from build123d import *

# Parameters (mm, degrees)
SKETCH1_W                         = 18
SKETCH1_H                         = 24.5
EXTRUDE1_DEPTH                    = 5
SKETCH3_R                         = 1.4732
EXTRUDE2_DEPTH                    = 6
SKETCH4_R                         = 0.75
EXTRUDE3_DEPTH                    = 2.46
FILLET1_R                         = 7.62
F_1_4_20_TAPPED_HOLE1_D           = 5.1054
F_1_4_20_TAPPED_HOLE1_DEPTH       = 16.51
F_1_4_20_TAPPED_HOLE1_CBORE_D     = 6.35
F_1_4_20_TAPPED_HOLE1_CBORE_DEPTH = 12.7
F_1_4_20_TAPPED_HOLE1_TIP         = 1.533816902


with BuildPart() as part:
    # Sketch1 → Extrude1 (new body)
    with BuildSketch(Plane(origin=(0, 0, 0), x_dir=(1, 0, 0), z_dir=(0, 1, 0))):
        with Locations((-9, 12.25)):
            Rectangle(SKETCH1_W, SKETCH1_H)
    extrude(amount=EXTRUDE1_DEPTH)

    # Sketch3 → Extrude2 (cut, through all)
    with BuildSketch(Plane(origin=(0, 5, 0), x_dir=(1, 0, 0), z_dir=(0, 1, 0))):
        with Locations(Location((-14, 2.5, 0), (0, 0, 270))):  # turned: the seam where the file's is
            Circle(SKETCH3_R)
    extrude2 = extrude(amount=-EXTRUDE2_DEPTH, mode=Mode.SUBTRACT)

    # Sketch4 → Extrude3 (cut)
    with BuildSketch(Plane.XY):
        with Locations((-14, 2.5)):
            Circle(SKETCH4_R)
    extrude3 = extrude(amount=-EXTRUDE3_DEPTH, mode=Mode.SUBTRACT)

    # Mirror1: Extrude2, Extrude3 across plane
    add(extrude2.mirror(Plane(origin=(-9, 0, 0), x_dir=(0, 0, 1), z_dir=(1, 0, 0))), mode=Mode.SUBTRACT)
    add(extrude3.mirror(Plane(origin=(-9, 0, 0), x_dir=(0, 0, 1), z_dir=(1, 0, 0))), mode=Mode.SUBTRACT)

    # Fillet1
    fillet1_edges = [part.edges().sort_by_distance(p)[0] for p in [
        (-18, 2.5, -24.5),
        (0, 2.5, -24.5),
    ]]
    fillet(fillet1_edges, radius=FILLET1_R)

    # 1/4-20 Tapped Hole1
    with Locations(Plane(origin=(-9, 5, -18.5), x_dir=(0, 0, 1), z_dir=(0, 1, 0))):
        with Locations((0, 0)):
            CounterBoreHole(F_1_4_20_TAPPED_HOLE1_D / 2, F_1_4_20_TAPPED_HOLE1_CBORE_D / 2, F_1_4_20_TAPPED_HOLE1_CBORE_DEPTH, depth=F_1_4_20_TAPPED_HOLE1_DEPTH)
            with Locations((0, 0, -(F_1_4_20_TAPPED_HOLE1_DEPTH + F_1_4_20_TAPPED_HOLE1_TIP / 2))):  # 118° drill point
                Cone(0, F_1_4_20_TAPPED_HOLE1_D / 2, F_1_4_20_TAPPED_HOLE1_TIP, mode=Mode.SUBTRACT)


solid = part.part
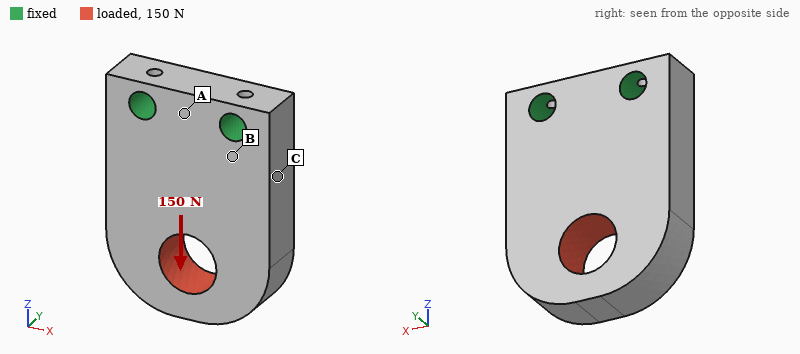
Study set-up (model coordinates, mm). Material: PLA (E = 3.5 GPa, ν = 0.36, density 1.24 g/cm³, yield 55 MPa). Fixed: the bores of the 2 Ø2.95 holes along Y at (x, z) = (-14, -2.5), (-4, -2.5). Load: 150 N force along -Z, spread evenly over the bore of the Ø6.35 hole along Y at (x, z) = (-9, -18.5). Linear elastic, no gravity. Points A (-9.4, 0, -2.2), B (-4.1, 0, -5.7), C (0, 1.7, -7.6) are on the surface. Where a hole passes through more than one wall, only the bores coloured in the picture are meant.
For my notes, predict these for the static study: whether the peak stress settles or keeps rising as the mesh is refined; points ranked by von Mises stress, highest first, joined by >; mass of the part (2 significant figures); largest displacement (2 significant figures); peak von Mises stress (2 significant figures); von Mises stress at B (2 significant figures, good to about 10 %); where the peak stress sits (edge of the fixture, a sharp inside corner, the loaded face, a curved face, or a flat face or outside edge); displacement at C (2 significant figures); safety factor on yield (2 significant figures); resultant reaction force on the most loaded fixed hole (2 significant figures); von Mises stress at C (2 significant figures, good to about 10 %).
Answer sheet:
settles
B > C > A
2.3 g
17 µm
5.5 MPa
2.4 MPa
the loaded face
3.5 µm
9.9
76 N
1.4 MPa
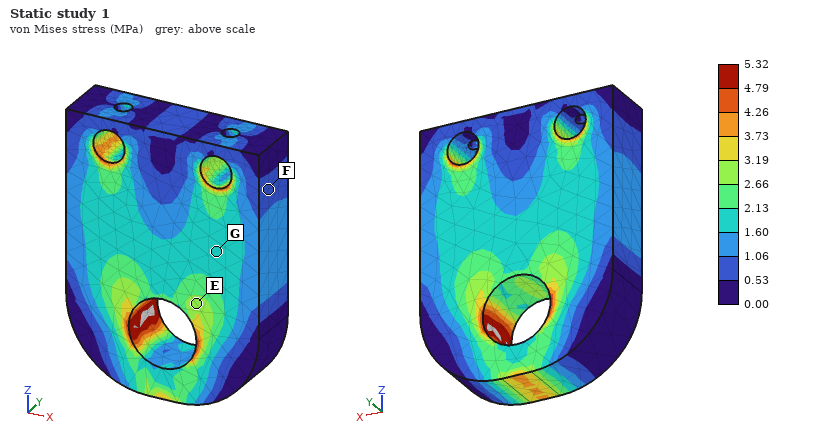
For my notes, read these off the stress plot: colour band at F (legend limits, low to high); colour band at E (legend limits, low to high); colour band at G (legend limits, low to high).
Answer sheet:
0.53 to 1.06 MPa
2.66 to 3.19 MPa
1.60 to 2.13 MPa
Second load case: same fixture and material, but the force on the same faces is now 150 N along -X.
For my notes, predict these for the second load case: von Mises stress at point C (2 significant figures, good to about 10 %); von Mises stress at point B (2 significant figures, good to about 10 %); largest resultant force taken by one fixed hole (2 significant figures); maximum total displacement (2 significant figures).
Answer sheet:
5.3 MPa
6.2 MPa
210 N
79 µm
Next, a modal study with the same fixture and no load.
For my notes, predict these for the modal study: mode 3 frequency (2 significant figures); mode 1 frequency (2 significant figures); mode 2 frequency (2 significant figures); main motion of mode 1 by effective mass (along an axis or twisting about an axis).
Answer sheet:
7800 Hz
3400 Hz
7600 Hz
along Y
